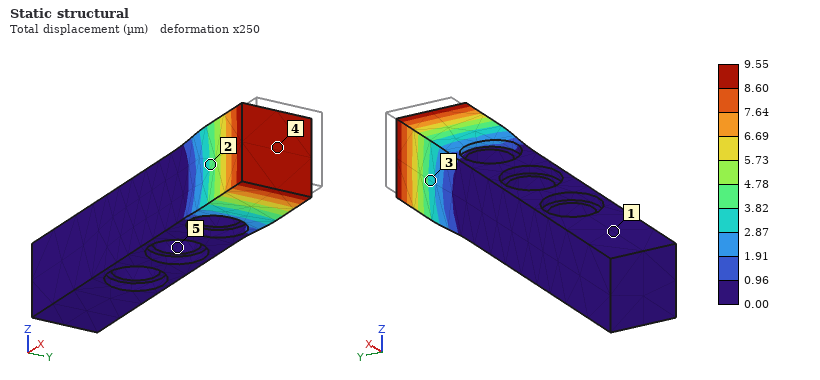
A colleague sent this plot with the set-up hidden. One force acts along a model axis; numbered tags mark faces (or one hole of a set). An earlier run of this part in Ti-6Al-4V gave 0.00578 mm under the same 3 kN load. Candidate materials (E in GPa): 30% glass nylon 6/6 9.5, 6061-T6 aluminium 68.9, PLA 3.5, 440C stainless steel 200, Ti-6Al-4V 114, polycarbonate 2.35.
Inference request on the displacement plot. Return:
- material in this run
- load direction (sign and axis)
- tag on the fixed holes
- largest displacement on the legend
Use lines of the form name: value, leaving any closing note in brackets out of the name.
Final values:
material in this run: 6061-T6 aluminium
load direction: -X
tag on the fixed holes: 5
largest displacement on the legend: 9.55 µm
